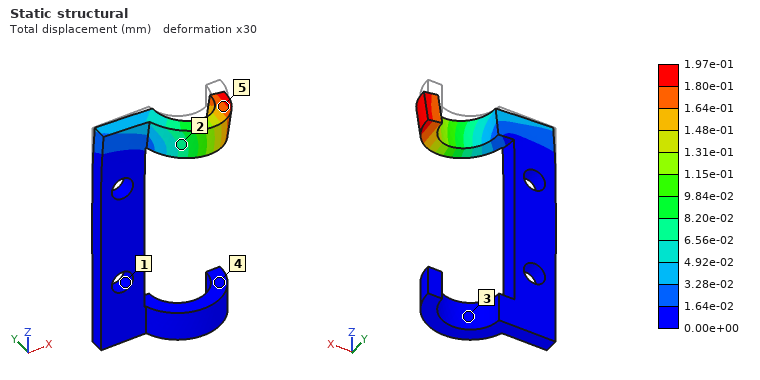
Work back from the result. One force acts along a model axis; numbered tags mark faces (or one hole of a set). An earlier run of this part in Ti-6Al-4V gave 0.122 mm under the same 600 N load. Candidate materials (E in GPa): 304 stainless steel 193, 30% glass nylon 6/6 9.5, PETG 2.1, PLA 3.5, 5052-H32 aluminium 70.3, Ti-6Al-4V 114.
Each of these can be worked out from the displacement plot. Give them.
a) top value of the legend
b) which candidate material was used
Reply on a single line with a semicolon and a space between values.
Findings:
1.97e-01 mm; 5052-H32 aluminium
